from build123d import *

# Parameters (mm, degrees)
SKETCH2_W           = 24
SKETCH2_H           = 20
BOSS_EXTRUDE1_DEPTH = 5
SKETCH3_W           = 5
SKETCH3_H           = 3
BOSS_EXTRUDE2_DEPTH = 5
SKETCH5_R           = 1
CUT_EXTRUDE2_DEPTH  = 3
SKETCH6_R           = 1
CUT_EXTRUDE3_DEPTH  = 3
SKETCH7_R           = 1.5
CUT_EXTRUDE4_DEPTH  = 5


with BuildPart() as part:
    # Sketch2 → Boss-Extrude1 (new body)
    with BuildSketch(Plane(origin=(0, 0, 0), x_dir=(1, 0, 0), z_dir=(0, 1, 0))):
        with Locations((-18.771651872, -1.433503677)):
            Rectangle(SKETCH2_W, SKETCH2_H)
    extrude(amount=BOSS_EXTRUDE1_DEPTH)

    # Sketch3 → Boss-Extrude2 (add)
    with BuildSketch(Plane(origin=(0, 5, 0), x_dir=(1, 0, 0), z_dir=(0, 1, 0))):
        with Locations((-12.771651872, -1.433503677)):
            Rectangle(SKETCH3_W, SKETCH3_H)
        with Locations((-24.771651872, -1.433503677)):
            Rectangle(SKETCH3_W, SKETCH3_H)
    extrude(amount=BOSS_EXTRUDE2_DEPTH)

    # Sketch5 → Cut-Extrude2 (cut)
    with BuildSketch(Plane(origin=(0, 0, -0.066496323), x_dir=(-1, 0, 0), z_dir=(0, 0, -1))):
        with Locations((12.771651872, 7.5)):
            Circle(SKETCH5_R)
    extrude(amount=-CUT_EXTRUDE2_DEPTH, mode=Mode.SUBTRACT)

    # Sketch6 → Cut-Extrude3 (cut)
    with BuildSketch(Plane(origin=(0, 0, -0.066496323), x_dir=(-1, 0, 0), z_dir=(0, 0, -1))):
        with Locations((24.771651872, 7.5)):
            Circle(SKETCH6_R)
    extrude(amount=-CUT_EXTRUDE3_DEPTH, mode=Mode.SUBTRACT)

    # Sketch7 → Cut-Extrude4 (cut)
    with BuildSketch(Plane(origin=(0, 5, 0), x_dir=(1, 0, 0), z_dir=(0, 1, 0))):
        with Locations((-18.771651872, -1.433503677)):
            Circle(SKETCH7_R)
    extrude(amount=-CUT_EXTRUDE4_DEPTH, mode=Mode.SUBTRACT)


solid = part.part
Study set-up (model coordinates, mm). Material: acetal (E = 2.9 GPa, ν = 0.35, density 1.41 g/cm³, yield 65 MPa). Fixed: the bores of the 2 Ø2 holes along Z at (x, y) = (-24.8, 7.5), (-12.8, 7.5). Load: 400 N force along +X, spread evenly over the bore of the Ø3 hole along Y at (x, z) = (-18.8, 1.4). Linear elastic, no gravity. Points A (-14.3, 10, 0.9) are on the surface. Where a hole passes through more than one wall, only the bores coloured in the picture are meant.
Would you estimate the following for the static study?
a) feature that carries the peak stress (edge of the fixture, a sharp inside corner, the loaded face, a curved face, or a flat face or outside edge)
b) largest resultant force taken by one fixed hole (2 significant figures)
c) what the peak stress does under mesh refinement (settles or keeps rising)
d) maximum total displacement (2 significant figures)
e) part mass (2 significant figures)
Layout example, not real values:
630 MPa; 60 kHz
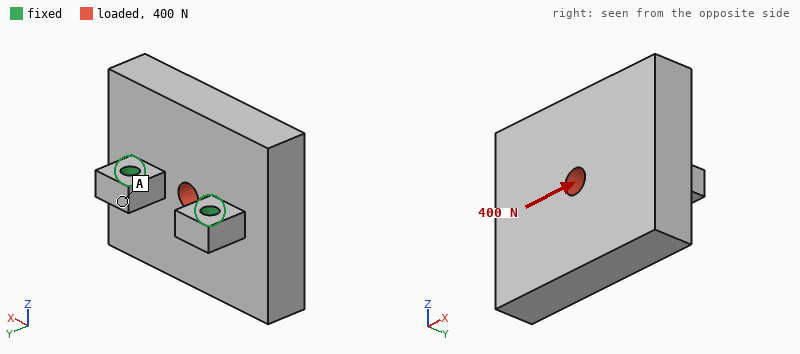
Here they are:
edge of the fixture; 230 N; keeps rising; 78 µm; 3.5 g
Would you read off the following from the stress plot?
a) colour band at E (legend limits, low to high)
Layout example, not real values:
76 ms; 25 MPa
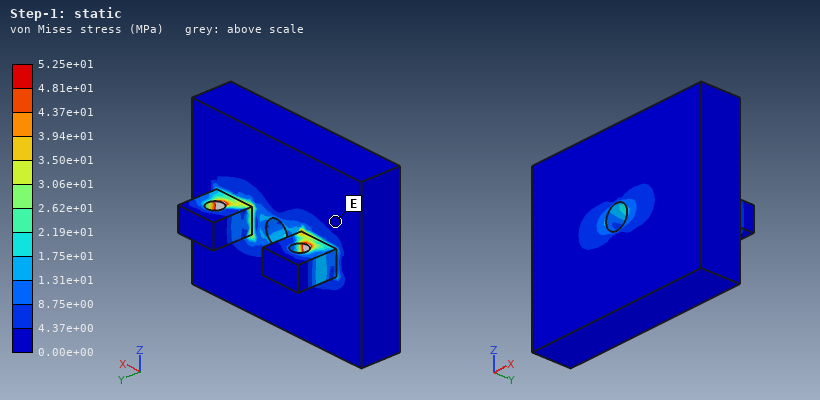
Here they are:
0.00e+00 to 4.37e+00 MPa
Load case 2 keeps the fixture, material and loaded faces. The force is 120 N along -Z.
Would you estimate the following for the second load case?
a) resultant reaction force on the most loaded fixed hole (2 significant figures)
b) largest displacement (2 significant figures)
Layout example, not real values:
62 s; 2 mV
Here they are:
60 N; 0.21 mm
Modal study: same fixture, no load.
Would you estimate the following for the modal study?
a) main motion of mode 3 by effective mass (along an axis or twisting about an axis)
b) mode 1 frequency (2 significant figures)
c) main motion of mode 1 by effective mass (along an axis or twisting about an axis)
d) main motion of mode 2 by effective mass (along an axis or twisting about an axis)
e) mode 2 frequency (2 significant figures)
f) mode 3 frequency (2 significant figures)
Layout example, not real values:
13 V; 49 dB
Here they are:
along X; 1900 Hz; along Z; twisting about Y; 4600 Hz; 6400 Hz
